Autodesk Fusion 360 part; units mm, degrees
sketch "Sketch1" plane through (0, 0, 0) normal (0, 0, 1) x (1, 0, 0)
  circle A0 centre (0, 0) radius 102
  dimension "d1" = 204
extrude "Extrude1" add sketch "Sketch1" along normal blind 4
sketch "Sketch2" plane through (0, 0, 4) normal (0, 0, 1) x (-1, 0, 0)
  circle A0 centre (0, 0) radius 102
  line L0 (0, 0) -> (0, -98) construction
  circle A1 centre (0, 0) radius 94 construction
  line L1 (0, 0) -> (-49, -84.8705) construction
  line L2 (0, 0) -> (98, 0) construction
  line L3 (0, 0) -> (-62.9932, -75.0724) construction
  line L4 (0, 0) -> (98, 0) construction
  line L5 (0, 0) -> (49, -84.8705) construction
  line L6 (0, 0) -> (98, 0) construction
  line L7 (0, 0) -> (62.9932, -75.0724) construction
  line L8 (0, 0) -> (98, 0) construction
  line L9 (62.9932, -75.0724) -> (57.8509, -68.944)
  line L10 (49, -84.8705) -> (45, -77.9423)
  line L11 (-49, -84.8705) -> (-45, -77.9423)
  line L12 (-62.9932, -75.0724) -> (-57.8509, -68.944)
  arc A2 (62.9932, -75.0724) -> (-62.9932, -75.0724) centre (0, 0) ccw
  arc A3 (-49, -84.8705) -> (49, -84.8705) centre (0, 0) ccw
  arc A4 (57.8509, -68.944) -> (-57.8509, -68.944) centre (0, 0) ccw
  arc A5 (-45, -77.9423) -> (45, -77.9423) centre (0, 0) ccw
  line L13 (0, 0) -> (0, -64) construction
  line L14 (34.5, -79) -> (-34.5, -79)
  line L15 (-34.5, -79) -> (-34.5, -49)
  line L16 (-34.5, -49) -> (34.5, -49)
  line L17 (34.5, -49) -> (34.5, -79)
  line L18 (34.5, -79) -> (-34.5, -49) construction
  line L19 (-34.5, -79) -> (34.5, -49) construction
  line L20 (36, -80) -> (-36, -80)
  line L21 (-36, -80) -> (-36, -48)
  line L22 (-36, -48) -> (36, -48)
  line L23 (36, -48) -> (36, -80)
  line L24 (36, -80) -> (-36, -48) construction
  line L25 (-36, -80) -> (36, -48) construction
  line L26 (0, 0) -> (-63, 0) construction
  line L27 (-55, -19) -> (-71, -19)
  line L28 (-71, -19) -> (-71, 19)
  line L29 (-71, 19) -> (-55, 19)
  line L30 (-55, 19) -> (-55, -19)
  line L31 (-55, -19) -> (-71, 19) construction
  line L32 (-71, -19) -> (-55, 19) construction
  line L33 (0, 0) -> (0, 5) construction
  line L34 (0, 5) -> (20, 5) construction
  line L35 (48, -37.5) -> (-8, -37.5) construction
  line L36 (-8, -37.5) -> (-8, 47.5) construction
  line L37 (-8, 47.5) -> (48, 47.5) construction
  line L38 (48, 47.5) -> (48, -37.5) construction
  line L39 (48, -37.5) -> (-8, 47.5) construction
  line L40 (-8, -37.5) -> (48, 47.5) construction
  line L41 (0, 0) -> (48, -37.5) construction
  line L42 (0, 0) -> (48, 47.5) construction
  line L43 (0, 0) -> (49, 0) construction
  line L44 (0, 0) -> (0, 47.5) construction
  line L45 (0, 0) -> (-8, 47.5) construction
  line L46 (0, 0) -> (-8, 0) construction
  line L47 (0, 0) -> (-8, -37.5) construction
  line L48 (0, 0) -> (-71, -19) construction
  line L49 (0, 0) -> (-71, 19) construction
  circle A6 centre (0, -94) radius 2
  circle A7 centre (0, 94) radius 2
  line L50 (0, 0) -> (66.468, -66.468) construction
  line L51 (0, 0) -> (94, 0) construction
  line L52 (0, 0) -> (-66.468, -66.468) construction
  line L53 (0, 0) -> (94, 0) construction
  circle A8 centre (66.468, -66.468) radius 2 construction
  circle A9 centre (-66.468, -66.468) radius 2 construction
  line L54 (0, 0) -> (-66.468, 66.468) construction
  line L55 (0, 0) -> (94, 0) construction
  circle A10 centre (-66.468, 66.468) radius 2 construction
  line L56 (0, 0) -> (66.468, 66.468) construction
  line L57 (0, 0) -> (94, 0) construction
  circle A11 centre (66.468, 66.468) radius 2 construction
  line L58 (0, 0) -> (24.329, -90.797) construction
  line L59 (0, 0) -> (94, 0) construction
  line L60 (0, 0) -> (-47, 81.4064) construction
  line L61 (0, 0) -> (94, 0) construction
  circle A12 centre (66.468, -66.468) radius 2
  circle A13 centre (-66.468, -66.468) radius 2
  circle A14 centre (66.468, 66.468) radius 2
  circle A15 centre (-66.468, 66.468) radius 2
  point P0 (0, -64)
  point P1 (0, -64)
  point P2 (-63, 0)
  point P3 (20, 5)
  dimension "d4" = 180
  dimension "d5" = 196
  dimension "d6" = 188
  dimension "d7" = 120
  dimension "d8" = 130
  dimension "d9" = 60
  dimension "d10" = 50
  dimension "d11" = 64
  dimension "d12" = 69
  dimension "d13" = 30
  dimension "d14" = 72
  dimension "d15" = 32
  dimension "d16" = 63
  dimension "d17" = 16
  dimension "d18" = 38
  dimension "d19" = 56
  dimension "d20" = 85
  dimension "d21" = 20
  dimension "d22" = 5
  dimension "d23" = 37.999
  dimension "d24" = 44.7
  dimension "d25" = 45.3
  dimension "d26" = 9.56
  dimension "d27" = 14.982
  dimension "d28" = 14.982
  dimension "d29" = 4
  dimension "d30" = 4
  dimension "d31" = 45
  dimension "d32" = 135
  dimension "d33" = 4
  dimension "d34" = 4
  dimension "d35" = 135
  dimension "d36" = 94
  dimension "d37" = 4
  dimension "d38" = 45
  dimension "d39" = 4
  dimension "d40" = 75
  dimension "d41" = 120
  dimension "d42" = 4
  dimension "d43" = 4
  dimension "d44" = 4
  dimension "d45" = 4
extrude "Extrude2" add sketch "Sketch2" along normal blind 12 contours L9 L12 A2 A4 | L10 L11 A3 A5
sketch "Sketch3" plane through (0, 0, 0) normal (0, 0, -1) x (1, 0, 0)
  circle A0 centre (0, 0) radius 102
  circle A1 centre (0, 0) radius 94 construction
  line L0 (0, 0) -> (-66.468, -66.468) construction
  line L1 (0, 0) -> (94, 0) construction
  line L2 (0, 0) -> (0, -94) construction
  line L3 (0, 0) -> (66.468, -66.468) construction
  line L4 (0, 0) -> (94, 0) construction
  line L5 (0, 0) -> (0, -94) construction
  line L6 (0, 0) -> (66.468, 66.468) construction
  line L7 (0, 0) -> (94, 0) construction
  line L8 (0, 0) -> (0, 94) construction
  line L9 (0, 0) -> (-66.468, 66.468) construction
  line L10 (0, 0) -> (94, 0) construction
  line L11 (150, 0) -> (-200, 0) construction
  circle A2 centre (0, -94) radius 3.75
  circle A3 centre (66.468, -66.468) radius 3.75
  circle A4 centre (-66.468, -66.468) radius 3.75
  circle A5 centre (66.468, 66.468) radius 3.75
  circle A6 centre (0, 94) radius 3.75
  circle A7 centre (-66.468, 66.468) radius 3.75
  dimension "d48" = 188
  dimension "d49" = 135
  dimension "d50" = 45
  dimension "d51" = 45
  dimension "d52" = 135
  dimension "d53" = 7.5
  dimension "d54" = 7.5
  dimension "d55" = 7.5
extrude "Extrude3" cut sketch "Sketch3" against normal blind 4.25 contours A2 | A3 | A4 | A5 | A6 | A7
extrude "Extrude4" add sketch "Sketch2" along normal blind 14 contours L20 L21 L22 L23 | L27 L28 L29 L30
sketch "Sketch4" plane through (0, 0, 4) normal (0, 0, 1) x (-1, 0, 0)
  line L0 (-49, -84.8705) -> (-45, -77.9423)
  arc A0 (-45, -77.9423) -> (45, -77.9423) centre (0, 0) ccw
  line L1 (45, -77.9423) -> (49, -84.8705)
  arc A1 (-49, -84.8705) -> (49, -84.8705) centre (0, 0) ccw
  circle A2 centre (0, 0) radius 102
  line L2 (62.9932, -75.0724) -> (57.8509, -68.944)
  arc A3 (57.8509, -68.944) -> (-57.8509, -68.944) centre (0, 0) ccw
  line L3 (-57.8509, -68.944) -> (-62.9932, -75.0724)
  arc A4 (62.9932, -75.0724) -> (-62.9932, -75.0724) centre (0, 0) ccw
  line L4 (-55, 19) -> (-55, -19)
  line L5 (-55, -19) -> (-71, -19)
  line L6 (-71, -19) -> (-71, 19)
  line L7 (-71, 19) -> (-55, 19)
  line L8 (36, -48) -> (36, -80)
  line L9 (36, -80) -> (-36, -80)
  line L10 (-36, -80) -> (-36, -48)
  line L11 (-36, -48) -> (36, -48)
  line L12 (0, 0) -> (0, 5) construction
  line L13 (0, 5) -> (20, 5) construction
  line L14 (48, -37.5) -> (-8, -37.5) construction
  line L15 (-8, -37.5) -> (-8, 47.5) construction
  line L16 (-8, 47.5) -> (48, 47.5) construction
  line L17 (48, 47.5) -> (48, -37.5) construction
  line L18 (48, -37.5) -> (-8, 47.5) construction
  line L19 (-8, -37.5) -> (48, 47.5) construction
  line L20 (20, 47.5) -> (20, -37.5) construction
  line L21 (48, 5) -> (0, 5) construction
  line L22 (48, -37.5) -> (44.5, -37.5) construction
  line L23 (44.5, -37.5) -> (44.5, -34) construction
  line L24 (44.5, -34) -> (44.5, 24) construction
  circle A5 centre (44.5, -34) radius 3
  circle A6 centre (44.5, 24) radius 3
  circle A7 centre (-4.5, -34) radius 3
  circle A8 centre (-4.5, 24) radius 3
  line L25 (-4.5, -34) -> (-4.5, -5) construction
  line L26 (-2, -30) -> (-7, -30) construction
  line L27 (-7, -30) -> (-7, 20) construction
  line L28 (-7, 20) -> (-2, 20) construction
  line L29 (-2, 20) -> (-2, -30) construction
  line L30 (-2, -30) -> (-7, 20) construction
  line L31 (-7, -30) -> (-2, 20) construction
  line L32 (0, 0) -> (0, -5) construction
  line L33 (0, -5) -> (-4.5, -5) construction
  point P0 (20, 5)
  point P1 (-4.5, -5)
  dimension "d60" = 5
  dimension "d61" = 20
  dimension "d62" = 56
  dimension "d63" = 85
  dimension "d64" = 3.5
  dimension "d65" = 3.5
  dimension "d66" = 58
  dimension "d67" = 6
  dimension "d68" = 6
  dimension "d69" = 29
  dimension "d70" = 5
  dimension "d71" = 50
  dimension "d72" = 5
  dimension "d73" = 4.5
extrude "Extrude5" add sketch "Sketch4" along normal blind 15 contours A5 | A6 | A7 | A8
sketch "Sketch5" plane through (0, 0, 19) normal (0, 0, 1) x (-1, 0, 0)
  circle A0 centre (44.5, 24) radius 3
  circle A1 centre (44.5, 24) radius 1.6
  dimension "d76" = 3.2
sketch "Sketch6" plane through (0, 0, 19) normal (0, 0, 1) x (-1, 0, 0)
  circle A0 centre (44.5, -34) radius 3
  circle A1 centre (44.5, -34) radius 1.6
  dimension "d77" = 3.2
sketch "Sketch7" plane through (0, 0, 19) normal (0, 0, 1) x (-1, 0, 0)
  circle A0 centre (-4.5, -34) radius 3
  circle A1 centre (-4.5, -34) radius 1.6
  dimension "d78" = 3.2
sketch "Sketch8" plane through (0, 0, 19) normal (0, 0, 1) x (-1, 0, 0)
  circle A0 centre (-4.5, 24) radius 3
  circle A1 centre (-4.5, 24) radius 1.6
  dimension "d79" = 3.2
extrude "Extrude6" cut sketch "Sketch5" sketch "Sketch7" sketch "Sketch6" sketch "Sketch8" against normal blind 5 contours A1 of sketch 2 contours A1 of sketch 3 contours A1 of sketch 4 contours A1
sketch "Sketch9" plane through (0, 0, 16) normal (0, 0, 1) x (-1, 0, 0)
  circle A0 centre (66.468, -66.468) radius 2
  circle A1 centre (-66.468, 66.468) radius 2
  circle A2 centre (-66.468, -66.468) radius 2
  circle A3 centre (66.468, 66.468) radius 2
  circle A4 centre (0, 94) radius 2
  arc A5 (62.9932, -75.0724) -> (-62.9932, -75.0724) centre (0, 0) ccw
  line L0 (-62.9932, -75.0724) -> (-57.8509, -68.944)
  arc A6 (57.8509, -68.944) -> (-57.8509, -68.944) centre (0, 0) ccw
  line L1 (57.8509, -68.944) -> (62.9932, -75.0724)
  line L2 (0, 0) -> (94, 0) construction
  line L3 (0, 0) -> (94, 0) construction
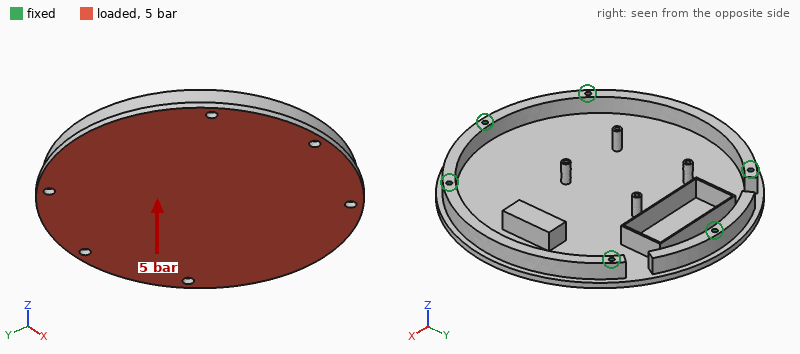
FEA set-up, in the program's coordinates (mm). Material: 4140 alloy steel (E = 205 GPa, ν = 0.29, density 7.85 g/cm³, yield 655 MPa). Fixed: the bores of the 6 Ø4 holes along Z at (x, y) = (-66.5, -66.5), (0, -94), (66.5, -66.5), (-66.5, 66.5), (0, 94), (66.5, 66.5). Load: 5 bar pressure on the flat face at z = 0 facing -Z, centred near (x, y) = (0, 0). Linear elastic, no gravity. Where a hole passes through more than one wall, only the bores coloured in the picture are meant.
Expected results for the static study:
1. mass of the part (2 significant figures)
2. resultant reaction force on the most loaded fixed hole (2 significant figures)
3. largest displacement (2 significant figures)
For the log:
1.5 kg
4.2 kN
0.49 mm
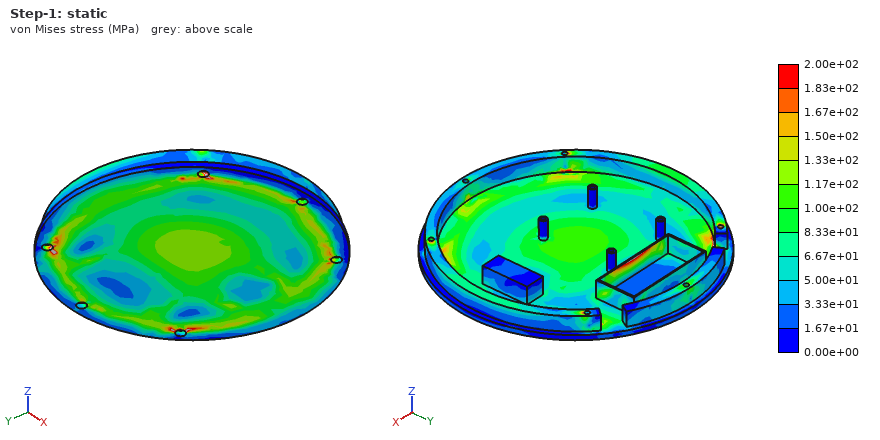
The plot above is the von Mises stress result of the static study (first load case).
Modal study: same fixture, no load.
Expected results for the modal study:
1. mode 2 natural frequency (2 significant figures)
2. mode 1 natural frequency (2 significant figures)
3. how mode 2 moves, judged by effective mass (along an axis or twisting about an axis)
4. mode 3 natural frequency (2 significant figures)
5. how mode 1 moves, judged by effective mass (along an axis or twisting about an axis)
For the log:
2000 Hz
1100 Hz
twisting about Y
2300 Hz
along Z
